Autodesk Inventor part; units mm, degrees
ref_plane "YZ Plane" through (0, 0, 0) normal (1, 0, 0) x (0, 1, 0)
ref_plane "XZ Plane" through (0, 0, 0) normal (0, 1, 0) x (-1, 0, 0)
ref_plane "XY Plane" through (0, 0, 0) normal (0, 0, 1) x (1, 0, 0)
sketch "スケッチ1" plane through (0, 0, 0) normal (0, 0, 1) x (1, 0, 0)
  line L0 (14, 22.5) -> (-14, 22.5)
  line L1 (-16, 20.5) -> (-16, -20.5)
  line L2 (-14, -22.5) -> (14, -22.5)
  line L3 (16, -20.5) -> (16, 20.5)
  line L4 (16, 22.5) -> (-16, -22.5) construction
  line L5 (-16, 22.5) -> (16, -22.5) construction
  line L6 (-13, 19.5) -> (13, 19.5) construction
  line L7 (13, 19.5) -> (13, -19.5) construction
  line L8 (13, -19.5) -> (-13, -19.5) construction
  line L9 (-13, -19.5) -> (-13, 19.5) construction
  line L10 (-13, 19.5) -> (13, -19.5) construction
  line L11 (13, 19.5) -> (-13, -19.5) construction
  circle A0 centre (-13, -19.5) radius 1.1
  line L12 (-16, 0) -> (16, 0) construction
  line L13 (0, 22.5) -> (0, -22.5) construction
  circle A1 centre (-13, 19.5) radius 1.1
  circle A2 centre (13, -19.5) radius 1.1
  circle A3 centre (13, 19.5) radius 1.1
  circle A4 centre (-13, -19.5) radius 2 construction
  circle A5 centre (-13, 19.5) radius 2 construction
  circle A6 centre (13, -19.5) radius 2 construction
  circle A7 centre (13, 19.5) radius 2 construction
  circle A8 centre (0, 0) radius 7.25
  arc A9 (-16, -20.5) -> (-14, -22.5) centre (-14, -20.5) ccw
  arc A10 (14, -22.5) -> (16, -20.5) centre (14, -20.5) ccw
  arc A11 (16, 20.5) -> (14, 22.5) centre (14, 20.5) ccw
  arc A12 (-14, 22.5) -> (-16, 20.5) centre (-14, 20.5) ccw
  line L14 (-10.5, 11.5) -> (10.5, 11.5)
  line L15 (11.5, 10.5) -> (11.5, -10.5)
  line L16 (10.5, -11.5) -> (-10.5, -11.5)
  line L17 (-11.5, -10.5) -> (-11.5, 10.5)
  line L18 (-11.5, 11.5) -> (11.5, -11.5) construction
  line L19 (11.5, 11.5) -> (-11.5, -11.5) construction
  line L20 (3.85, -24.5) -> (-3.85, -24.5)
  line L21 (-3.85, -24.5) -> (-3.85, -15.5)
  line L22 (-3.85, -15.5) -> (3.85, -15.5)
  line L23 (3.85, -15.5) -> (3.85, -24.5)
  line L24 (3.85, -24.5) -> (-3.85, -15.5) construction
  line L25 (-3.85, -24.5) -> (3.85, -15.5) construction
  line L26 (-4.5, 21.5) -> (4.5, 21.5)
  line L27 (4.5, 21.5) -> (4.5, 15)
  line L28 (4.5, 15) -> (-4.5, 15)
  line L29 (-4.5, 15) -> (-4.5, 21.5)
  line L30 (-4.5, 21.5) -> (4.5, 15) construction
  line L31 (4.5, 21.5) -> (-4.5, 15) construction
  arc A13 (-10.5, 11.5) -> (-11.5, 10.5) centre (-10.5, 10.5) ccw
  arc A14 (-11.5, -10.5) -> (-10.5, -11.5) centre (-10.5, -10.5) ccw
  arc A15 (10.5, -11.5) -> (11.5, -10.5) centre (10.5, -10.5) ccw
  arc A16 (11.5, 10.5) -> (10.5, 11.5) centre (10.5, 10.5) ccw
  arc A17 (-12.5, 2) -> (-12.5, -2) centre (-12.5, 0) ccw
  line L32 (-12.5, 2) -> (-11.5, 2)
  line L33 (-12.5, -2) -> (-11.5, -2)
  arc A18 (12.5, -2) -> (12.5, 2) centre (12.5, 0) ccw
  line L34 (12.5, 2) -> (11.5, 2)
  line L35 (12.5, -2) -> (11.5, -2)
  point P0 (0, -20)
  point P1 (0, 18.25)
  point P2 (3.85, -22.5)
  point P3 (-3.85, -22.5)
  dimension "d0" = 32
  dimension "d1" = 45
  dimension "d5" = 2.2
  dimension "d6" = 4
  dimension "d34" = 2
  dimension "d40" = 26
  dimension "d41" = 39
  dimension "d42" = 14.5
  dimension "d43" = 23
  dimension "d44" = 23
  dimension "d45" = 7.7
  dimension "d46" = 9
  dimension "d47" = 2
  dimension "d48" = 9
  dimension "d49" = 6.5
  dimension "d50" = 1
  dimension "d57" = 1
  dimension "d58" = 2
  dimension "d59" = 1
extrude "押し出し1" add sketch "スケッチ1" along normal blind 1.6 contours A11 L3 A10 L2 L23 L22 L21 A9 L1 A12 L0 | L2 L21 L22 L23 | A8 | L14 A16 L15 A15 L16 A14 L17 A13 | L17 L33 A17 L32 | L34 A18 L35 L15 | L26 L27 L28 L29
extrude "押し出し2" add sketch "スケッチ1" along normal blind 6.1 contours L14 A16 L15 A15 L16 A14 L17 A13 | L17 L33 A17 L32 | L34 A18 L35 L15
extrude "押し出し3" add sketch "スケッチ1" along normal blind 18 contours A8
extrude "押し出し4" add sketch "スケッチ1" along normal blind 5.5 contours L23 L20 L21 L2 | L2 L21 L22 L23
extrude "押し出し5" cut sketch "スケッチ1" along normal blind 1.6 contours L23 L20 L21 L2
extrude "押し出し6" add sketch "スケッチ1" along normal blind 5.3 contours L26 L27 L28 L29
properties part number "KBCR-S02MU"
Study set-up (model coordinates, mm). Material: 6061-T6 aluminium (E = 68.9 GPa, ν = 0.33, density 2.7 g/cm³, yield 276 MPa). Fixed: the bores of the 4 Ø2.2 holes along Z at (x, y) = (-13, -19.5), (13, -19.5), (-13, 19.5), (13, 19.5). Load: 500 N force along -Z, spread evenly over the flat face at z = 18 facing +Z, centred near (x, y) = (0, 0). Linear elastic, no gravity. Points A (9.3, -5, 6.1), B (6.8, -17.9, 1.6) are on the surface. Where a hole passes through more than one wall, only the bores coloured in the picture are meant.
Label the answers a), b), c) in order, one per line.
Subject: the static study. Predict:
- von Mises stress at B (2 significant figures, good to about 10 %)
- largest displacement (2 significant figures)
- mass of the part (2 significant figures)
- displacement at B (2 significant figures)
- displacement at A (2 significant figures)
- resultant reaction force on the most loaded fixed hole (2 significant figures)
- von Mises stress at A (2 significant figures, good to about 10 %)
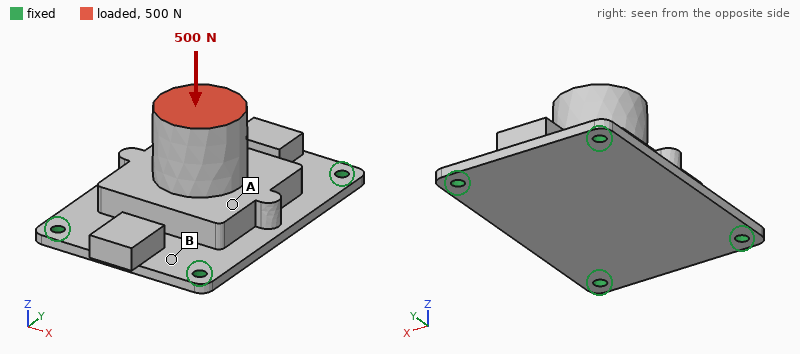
a) 23 MPa
b) 43 µm
c) 19 g
d) 15 µm
e) 41 µm
f) 160 N
g) 13 MPa
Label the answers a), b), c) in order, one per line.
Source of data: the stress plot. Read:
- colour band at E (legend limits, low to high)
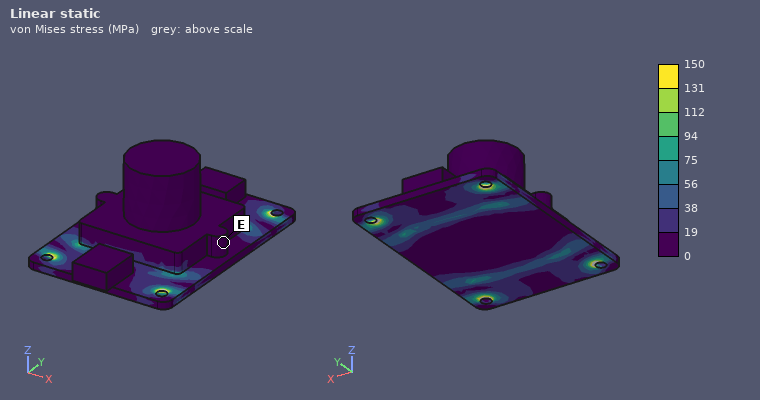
a) 0 to 19 MPa
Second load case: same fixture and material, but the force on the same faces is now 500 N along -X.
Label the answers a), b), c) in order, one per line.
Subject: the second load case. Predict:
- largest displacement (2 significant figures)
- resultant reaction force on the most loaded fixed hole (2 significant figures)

a) 0.10 mm
b) 270 N
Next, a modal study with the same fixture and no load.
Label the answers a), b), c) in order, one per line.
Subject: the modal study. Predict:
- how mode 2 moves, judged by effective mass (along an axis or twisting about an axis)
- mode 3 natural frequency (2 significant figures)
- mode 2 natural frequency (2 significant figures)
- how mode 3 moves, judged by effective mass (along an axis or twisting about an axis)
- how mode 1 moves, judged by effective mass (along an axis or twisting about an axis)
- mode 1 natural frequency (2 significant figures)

a) along X
b) 7200 Hz
c) 5300 Hz
d) along Y
e) along Z
f) 4400 Hz
